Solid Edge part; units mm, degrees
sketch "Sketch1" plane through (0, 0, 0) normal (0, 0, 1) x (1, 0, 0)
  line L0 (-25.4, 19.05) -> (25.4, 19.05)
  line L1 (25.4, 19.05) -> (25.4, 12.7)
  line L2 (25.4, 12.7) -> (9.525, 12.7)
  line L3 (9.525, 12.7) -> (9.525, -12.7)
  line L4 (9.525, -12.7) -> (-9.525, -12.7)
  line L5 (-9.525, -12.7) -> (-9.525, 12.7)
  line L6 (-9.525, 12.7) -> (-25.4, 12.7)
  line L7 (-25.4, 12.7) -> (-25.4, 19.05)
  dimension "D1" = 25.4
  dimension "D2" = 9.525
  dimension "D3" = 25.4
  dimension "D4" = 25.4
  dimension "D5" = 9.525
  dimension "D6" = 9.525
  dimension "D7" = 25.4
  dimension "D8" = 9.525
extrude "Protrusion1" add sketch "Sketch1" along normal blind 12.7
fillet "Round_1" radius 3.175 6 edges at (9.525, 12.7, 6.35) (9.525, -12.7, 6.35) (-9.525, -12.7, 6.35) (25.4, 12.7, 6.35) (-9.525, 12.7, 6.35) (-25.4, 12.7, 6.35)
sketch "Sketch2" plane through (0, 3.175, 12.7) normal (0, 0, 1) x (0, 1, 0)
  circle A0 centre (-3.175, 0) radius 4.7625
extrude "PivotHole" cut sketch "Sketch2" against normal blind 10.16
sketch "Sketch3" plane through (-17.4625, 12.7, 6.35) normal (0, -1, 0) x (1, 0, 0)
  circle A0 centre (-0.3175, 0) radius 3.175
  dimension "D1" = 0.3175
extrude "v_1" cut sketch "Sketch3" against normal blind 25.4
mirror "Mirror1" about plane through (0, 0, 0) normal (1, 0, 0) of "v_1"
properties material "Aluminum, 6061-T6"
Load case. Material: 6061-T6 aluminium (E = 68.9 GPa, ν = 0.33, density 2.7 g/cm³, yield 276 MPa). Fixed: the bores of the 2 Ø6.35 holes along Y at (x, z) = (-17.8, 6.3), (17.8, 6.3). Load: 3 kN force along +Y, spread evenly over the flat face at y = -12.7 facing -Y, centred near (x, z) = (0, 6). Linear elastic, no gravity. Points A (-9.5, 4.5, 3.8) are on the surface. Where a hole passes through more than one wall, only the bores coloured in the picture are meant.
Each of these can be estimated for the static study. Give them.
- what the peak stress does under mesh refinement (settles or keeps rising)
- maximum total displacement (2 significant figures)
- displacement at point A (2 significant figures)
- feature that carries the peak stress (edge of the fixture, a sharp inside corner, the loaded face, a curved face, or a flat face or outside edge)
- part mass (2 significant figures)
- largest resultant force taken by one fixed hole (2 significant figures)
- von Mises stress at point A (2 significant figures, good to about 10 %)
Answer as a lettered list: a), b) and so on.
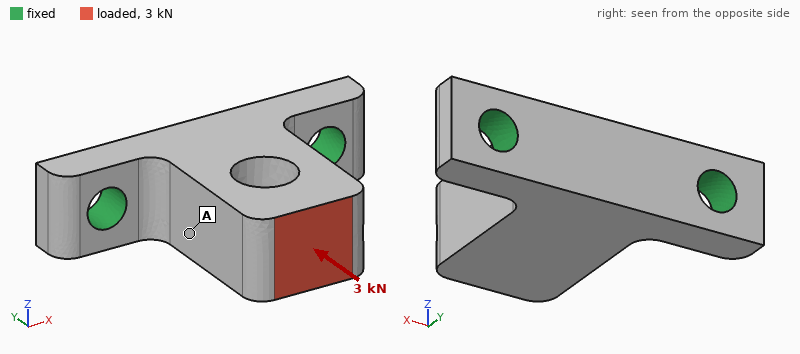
a) keeps rising
b) 20 µm
c) 12 µm
d) edge of the fixture
e) 24 g
f) 1.6 kN
g) 19 MPa
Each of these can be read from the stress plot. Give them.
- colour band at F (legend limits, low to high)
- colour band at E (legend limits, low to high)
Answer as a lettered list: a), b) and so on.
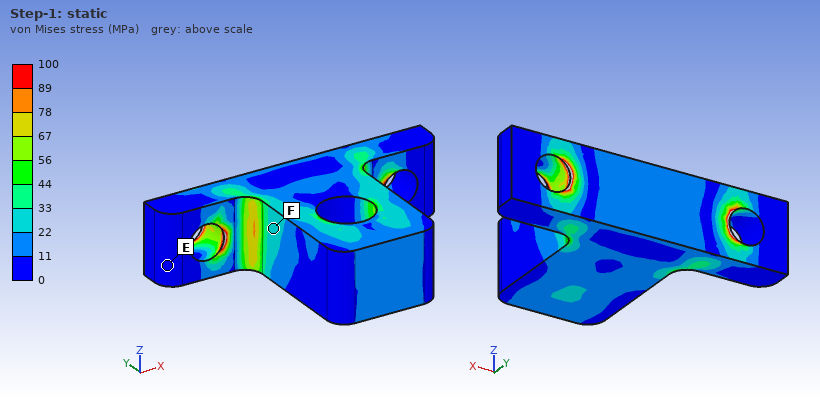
a) 22 to 33 MPa
b) 0 to 11 MPa
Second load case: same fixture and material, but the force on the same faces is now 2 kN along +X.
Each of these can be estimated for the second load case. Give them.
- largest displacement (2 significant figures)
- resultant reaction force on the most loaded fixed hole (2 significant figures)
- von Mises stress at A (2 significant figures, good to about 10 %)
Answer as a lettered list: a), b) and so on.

a) 71 µm
b) 2.4 kN
c) 63 MPa
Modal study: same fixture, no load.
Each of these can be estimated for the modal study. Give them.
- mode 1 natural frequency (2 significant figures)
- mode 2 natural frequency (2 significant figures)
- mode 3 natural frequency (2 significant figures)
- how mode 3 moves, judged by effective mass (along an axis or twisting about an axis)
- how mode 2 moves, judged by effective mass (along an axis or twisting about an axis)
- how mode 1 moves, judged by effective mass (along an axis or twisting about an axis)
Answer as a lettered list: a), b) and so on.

a) 5300 Hz
b) 12 kHz
c) 19 kHz
d) along Y
e) along X
f) along Z
